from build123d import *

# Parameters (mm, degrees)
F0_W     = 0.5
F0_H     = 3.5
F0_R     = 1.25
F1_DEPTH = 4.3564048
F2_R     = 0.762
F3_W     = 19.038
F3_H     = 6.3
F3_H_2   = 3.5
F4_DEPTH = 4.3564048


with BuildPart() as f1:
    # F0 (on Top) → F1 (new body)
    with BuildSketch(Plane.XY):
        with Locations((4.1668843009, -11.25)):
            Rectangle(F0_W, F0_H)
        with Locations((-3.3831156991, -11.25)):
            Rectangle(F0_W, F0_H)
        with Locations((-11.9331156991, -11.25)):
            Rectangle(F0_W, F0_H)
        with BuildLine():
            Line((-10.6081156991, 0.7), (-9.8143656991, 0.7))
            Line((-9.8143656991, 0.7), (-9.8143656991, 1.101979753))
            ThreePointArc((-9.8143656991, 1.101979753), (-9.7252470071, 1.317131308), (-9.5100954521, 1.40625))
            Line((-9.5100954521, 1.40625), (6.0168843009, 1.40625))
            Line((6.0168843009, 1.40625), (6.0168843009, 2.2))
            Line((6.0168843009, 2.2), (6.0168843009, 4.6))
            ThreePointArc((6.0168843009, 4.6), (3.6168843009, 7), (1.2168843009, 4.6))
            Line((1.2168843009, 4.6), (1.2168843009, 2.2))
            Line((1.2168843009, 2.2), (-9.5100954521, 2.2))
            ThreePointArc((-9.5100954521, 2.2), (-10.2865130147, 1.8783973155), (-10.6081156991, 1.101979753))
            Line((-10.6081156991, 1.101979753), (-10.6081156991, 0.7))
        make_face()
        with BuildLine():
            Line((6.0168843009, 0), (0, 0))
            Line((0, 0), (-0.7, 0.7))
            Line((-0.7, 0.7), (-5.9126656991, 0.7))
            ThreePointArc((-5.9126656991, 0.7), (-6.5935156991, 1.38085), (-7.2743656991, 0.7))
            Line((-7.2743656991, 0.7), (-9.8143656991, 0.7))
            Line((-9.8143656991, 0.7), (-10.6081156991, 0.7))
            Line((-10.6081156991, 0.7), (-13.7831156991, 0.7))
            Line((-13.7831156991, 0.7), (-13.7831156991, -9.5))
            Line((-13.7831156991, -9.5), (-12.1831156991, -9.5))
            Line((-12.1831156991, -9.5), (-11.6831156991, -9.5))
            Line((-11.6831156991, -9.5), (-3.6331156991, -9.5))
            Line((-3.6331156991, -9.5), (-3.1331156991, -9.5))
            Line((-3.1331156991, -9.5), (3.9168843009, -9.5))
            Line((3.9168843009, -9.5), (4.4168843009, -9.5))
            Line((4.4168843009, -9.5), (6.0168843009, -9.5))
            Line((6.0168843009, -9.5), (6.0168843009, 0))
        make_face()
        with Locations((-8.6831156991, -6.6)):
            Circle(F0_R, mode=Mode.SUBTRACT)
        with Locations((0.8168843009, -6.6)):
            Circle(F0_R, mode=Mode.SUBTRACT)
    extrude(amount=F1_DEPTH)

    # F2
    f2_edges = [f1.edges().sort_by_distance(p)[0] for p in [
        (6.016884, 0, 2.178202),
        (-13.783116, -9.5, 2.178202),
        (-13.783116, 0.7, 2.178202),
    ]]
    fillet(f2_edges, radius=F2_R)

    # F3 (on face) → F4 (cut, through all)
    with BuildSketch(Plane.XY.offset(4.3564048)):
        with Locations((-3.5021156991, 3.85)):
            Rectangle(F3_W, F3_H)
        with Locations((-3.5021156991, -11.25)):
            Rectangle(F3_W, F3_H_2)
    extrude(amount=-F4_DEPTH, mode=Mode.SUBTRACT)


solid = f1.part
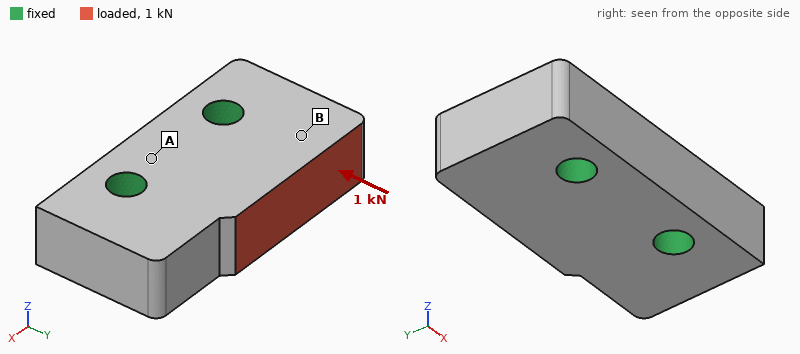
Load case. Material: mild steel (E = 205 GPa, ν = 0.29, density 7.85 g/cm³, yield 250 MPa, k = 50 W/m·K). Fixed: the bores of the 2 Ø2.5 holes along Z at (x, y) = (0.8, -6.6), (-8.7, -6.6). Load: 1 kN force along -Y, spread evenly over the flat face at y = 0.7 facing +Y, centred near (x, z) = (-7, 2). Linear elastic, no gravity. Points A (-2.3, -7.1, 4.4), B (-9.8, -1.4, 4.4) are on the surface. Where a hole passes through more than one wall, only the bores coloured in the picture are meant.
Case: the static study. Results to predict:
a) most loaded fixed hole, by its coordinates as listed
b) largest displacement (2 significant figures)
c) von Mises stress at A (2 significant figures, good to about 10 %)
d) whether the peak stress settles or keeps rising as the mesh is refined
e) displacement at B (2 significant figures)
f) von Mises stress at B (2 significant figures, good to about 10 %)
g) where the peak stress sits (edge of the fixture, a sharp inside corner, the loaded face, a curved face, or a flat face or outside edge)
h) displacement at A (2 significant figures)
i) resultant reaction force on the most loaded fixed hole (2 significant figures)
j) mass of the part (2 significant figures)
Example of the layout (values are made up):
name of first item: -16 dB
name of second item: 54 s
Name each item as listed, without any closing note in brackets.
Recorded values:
most loaded fixed hole, by its coordinates as listed: (-8.7, -6.6)
largest displacement: 0.95 µm
von Mises stress at A: 6.8 MPa
whether the peak stress settles or keeps rising as the mesh is refined: keeps rising
displacement at B: 0.66 µm
von Mises stress at B: 22 MPa
where the peak stress sits: edge of the fixture
displacement at A: 0.19 µm
resultant reaction force on the most loaded fixed hole: 770 N
mass of the part: 6.4 g
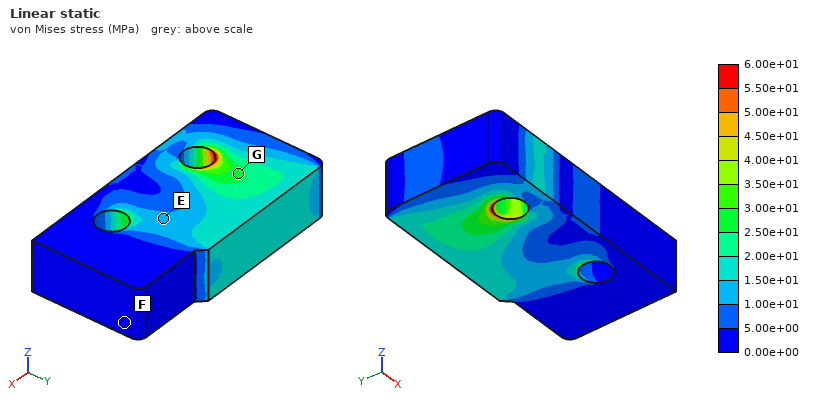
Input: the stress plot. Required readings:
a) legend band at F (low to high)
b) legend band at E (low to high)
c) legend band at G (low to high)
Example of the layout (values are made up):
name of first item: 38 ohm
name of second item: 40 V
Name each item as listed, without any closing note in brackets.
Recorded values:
legend band at F: 0.00e+00 to 5.00e+00 MPa
legend band at E: 1.00e+01 to 1.50e+01 MPa
legend band at G: 2.50e+01 to 3.00e+01 MPa
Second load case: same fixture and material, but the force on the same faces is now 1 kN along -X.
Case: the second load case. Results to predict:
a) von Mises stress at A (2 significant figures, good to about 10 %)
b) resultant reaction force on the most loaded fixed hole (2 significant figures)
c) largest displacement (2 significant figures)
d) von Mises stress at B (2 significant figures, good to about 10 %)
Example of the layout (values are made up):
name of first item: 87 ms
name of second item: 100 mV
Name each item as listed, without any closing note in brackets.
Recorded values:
von Mises stress at A: 9.8 MPa
resultant reaction force on the most loaded fixed hole: 780 N
largest displacement: 3.2 µm
von Mises stress at B: 25 MPa
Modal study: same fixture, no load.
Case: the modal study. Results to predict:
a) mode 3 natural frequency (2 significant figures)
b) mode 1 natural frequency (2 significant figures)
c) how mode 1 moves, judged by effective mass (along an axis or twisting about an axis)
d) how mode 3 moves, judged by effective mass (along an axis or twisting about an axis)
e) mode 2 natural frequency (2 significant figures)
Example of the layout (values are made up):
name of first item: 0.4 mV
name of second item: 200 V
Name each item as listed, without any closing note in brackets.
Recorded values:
mode 3 natural frequency: 76 kHz
mode 1 natural frequency: 55 kHz
how mode 1 moves, judged by effective mass: along Z
how mode 3 moves, judged by effective mass: along X
mode 2 natural frequency: 66 kHz
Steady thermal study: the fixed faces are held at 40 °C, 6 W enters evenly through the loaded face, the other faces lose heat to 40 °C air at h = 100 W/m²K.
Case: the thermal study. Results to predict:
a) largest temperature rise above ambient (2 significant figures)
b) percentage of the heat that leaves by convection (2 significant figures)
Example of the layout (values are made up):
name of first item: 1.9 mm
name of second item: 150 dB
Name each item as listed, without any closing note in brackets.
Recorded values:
largest temperature rise above ambient: 14 K
percentage of the heat that leaves by convection: 3.5 %
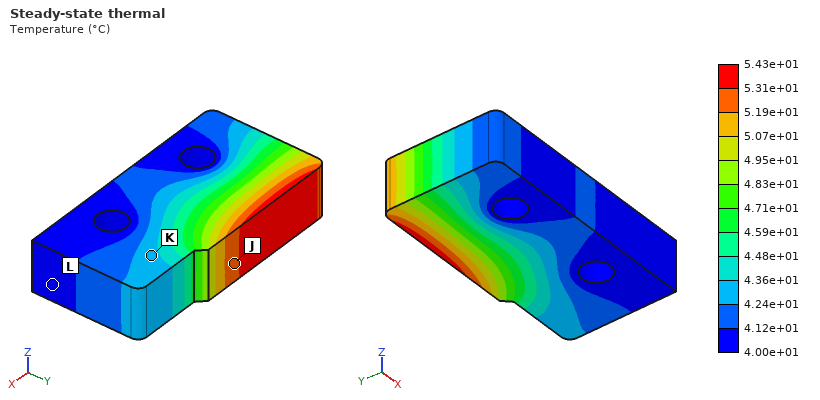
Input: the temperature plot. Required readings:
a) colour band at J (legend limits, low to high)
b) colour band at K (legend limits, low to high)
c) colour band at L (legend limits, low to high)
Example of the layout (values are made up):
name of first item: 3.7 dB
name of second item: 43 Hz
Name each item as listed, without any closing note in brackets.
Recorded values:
colour band at J: 5.19e+01 to 5.31e+01 °C
colour band at K: 4.24e+01 to 4.36e+01 °C
colour band at L: 4.00e+01 to 4.12e+01 °C
